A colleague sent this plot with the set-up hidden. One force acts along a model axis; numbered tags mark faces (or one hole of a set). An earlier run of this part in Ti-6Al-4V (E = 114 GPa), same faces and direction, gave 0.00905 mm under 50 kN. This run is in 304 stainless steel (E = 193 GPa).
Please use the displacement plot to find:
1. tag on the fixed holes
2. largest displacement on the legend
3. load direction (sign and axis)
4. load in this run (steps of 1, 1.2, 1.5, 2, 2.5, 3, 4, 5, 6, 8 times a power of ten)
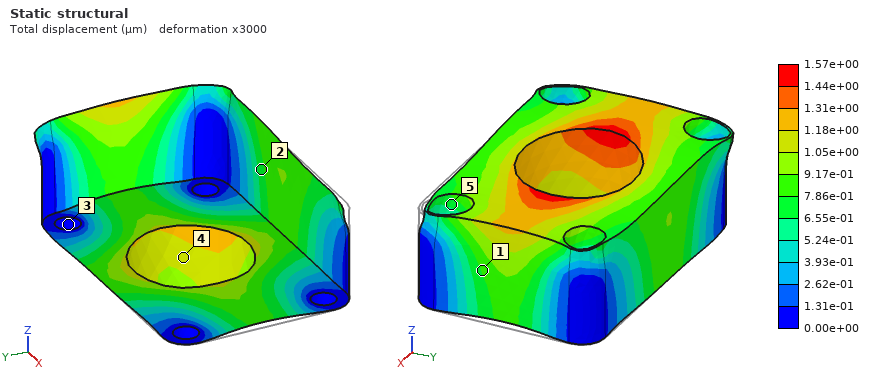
3
1.57e+00 µm
-X
15 kN
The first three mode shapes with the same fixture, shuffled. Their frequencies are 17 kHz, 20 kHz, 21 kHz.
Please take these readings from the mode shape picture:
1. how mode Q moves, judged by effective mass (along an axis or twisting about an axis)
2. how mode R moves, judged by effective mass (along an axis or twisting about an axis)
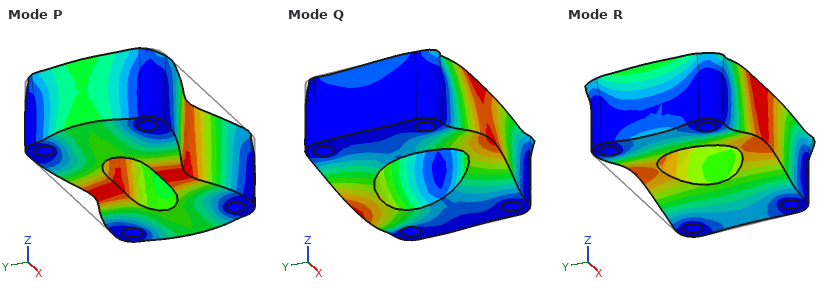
twisting about X
along Z
